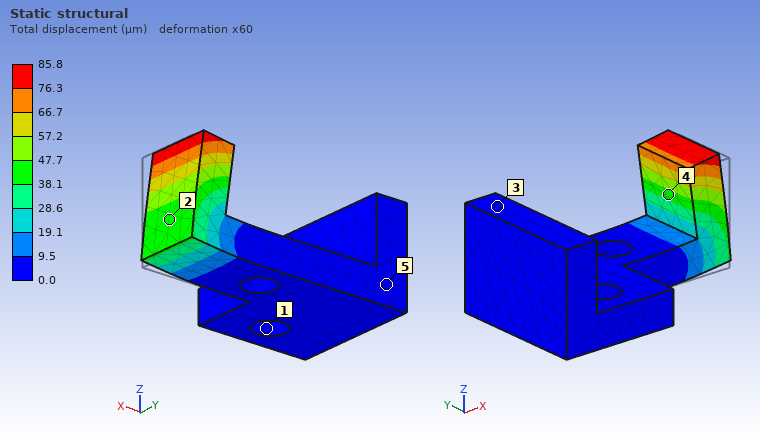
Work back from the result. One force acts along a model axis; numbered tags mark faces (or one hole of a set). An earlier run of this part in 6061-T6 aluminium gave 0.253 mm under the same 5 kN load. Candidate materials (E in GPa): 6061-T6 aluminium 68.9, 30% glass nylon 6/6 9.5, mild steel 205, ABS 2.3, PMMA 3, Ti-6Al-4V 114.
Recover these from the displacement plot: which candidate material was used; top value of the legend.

mild steel
85.8 µm
